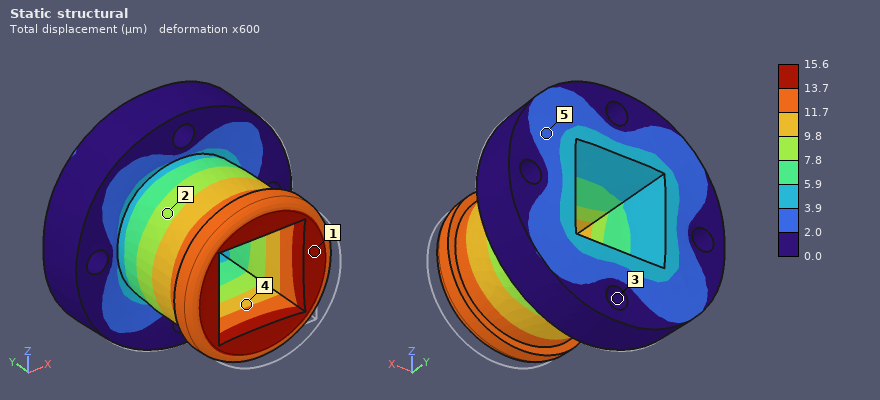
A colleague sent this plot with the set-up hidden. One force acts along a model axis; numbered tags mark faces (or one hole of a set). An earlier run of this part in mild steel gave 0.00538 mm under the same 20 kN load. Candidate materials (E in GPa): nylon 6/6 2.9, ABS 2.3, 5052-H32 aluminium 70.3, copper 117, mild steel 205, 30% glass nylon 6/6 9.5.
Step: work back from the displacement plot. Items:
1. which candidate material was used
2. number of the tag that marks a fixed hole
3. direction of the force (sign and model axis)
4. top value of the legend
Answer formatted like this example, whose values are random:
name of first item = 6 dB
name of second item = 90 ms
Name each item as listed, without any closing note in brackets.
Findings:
which candidate material was used = 5052-H32 aluminium
number of the tag that marks a fixed hole = 3
direction of the force = +Y
top value of the legend = 15.6 µm
